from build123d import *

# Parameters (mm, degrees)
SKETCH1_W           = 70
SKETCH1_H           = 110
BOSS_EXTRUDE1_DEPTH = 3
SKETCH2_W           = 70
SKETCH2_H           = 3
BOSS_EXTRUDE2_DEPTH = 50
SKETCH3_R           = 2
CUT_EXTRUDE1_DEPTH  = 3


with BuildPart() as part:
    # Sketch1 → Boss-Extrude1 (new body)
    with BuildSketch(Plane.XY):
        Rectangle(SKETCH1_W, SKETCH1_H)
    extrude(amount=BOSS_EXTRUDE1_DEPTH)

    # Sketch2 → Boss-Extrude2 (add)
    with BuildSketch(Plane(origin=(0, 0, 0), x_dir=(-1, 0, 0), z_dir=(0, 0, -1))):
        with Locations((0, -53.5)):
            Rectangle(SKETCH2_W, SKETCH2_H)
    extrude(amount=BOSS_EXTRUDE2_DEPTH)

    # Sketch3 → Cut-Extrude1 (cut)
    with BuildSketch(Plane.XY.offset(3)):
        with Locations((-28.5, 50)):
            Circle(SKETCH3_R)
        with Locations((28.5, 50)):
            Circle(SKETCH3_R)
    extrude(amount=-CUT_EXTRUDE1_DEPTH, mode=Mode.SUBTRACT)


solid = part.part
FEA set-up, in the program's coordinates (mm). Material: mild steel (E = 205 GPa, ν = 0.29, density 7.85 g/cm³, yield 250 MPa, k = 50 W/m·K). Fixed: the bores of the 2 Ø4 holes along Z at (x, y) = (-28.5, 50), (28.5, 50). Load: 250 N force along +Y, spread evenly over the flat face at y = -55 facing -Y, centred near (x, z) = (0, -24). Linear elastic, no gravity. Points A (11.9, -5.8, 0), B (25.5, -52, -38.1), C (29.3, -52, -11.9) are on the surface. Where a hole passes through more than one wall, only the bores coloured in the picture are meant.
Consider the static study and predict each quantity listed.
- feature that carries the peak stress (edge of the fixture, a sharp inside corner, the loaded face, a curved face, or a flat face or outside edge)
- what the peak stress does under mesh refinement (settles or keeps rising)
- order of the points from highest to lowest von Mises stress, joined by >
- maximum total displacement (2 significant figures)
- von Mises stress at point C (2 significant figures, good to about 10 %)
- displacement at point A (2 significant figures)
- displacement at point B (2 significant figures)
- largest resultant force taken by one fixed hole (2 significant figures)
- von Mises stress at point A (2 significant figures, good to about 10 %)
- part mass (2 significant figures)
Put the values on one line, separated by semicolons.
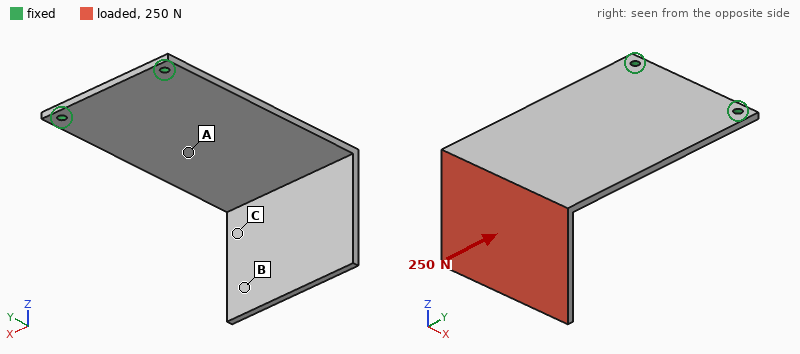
edge of the fixture; keeps rising; A > C > B; 1.7 mm; 29 MPa; 0.38 mm; 1.4 mm; 130 N; 58 MPa; 260 g
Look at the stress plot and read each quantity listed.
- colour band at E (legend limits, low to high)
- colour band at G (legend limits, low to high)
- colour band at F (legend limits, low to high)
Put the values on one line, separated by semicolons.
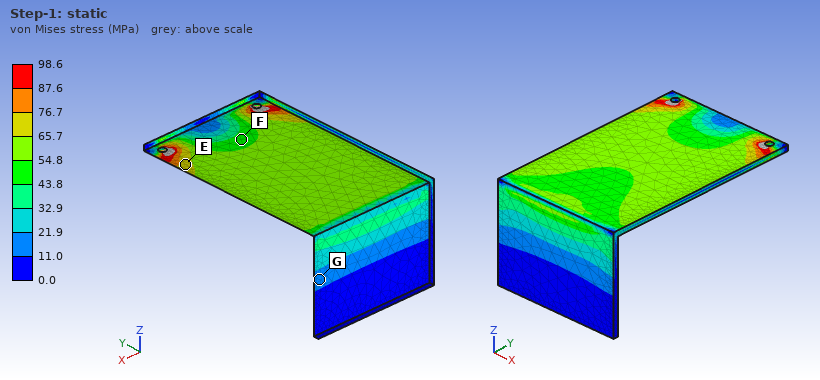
65.7 to 76.7 MPa; 11.0 to 21.9 MPa; 43.8 to 54.8 MPa
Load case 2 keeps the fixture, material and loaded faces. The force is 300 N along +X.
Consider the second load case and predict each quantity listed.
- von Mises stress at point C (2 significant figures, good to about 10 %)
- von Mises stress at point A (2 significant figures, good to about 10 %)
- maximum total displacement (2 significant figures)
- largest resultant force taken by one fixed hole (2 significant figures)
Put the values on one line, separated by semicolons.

24 MPa; 62 MPa; 0.75 mm; 580 N
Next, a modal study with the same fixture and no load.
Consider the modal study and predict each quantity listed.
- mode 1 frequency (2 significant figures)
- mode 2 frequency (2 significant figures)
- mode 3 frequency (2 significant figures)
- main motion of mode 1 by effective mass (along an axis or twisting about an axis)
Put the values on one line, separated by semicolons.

120 Hz; 340 Hz; 510 Hz; along Z
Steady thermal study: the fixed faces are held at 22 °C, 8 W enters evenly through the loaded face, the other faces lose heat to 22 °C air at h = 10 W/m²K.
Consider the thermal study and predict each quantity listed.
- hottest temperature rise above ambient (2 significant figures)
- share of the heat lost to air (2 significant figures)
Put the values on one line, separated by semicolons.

55 K; 64 %
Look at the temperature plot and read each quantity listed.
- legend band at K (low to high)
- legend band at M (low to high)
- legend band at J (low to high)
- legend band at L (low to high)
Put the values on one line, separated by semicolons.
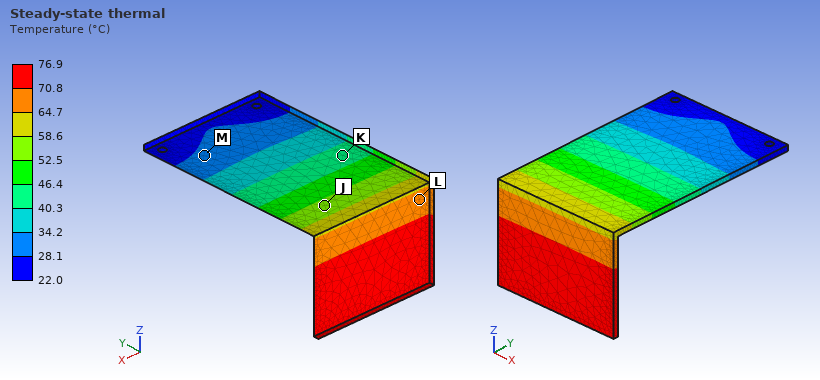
40.3 to 46.4 °C; 28.1 to 34.2 °C; 52.5 to 58.6 °C; 64.7 to 70.8 °C
